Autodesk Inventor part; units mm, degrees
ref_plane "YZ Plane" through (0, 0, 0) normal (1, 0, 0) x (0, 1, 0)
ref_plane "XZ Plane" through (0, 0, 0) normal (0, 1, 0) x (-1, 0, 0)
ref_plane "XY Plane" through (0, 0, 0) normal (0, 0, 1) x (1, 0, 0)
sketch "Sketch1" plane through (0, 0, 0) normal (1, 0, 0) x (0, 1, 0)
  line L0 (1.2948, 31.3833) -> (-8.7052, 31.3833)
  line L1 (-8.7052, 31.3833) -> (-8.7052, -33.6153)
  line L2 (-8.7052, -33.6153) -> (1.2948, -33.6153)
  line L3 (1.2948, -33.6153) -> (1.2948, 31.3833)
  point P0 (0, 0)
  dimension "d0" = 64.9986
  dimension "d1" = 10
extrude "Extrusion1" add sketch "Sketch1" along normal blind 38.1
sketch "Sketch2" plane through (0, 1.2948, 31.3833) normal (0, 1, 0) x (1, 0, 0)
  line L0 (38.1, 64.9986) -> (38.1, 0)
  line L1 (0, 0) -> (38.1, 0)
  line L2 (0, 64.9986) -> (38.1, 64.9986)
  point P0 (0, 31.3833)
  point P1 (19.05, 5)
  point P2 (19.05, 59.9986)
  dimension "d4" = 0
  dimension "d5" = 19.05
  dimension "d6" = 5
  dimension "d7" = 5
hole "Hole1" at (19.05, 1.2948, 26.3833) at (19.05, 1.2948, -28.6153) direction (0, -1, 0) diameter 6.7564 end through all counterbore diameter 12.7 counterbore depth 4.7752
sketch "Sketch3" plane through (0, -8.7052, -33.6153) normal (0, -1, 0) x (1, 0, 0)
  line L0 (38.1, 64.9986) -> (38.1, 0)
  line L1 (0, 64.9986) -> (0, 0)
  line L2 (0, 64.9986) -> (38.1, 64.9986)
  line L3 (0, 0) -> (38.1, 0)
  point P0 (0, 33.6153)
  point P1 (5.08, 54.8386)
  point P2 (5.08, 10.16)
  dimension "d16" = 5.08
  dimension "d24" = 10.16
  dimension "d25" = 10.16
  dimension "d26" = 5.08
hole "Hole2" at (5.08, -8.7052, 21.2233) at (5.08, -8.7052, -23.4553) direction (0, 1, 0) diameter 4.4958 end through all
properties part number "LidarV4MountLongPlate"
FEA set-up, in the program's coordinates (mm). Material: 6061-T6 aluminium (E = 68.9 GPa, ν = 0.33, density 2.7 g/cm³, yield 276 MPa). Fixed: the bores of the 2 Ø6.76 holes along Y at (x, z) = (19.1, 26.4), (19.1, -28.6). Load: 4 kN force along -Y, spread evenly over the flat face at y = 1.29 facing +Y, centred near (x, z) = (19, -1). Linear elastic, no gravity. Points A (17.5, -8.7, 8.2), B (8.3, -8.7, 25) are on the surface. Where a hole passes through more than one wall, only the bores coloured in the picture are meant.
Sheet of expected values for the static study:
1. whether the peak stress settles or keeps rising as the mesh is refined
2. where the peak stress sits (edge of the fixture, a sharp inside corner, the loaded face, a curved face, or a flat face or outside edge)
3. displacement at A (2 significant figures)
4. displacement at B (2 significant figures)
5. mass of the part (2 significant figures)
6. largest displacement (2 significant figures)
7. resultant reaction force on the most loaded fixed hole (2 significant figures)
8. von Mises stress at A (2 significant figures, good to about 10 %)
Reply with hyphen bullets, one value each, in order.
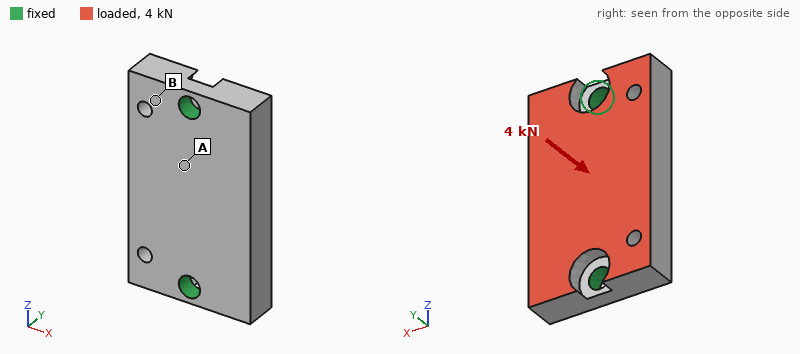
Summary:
- keeps rising
- edge of the fixture
- 18 µm
- 7.5 µm
- 62 g
- 28 µm
- 2.3 kN
- 17 MPa
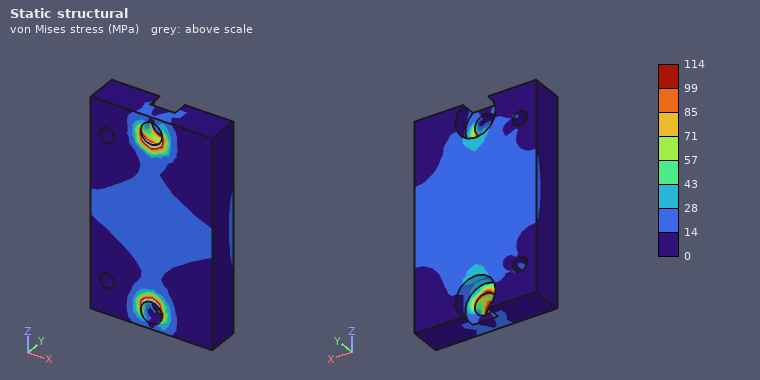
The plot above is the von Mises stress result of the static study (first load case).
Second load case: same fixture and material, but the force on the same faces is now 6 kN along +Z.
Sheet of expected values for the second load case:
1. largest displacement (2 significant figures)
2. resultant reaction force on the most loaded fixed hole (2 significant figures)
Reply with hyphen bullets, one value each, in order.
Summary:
- 9.5 µm
- 3.1 kN
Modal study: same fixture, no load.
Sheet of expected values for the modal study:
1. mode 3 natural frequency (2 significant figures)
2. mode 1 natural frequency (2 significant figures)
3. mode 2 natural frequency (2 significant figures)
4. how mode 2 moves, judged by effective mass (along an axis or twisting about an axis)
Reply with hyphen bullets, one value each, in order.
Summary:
- 15 kHz
- 6500 Hz
- 9400 Hz
- along Y
